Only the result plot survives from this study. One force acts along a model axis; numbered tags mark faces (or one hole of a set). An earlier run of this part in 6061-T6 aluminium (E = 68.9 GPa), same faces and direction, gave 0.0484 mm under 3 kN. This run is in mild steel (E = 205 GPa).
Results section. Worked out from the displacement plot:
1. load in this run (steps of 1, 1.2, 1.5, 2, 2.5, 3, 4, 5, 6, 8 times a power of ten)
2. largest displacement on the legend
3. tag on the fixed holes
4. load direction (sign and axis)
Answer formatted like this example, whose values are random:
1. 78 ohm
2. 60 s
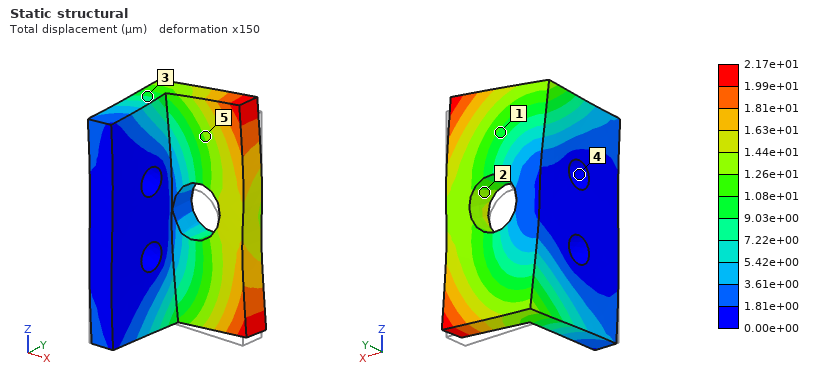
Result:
1. 4 kN
2. 2.17e+01 µm
3. 4
4. +Z
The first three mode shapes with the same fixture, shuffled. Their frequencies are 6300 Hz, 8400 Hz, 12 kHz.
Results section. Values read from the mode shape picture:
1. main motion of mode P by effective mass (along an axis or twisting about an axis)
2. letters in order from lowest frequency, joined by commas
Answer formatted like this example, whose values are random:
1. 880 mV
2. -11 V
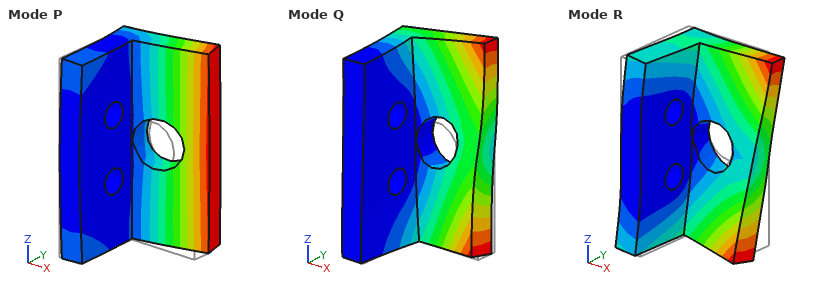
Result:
1. along Y
2. P, Q, R
